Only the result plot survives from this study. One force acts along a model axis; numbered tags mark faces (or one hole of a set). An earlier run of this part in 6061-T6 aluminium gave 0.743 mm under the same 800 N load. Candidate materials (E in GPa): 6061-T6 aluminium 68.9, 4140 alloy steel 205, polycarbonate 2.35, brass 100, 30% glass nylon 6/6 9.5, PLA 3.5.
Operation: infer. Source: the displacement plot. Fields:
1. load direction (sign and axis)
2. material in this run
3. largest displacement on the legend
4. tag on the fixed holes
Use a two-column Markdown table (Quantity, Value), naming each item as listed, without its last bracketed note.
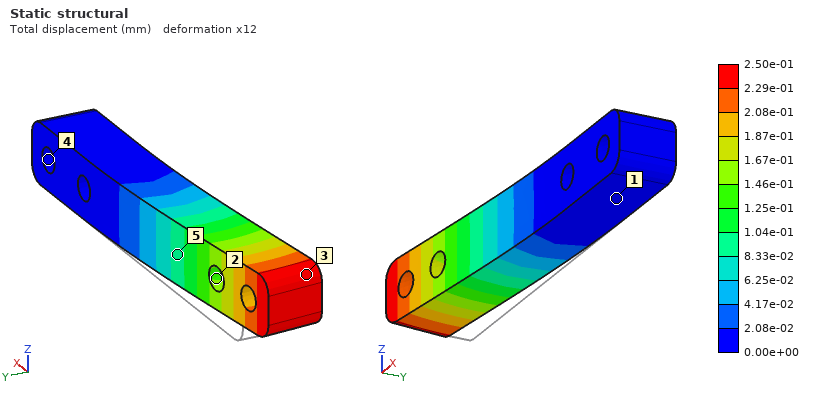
| Quantity | Value |
|---|---|
| load direction | -Y |
| material in this run | 4140 alloy steel |
| largest displacement on the legend | 2.50e-01 mm |
| tag on the fixed holes | 4 |
